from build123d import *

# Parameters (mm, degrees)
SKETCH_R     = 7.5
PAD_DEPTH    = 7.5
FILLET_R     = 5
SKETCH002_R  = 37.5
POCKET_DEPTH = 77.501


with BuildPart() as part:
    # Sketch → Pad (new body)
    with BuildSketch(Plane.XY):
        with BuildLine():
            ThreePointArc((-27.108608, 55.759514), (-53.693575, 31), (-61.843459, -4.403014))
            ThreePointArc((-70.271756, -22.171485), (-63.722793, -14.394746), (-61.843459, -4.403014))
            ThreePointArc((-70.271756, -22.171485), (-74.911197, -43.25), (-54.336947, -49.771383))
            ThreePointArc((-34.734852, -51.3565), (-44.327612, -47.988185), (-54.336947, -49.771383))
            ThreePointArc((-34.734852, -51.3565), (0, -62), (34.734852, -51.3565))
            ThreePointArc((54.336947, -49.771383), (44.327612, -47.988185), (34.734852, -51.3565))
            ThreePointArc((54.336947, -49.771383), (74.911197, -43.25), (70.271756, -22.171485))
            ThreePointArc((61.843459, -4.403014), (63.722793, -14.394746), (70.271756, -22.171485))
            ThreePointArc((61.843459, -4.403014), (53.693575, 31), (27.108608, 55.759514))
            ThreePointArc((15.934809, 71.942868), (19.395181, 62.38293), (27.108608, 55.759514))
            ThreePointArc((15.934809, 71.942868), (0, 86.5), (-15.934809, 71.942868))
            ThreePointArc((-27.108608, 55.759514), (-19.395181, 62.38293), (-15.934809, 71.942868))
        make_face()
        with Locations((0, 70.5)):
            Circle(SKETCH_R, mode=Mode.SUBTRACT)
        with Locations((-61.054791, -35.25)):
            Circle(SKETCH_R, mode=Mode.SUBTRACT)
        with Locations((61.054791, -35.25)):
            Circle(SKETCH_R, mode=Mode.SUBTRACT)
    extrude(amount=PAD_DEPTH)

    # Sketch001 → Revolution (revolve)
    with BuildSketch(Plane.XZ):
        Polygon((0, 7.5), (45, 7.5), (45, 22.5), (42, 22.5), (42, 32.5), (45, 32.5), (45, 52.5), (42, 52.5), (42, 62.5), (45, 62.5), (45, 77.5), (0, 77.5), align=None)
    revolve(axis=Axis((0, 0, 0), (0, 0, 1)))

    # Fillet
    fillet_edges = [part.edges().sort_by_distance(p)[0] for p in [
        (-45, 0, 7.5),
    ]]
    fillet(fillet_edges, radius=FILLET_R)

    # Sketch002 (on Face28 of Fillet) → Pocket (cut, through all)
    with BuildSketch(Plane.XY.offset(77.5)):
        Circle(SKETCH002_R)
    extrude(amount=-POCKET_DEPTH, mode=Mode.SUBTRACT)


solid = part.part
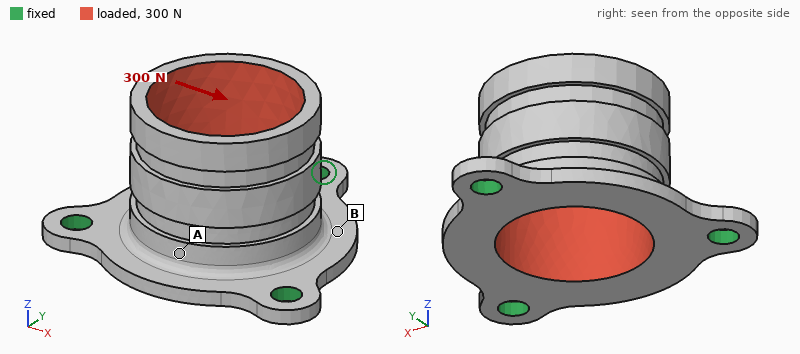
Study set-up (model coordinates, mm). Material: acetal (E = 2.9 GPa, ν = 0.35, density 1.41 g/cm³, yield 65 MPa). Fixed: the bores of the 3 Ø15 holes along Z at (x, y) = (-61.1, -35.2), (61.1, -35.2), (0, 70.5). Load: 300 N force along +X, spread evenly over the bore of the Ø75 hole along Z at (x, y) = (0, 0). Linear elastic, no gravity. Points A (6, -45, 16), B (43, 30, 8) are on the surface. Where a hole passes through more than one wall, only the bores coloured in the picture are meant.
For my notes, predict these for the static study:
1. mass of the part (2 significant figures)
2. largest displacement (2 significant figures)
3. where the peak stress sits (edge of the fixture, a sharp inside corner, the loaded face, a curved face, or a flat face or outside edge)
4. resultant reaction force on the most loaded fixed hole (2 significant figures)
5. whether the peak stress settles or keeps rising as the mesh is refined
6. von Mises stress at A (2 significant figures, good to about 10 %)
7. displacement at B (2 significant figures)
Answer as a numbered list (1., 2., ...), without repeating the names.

1. 270 g
2. 0.13 mm
3. edge of the fixture
4. 140 N
5. keeps rising
6. 0.39 MPa
7. 0.060 mm
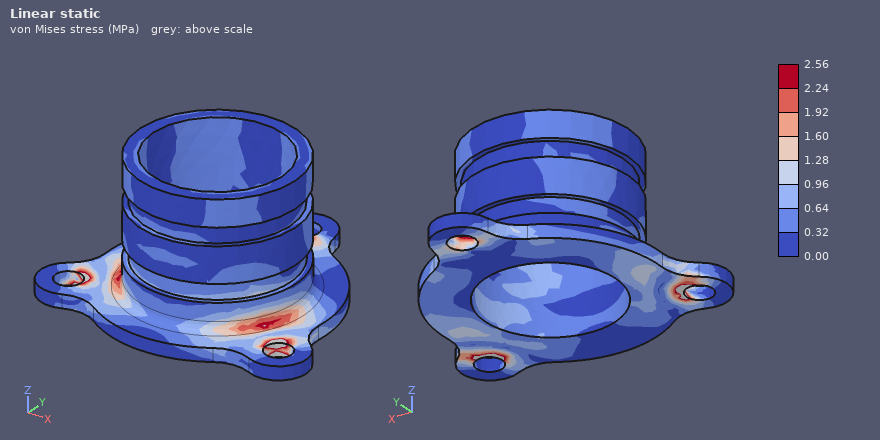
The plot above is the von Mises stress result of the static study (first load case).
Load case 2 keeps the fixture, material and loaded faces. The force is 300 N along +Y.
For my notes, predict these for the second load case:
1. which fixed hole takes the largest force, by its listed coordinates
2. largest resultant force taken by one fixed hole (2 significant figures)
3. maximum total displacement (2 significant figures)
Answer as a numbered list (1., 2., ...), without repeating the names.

1. (0, 70.5)
2. 160 N
3. 0.14 mm
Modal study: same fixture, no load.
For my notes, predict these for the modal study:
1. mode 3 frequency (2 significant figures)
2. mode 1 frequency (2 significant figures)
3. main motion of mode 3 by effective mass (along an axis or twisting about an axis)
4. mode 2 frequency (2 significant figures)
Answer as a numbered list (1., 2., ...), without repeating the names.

1. 830 Hz
2. 600 Hz
3. along Z
4. 600 Hz
